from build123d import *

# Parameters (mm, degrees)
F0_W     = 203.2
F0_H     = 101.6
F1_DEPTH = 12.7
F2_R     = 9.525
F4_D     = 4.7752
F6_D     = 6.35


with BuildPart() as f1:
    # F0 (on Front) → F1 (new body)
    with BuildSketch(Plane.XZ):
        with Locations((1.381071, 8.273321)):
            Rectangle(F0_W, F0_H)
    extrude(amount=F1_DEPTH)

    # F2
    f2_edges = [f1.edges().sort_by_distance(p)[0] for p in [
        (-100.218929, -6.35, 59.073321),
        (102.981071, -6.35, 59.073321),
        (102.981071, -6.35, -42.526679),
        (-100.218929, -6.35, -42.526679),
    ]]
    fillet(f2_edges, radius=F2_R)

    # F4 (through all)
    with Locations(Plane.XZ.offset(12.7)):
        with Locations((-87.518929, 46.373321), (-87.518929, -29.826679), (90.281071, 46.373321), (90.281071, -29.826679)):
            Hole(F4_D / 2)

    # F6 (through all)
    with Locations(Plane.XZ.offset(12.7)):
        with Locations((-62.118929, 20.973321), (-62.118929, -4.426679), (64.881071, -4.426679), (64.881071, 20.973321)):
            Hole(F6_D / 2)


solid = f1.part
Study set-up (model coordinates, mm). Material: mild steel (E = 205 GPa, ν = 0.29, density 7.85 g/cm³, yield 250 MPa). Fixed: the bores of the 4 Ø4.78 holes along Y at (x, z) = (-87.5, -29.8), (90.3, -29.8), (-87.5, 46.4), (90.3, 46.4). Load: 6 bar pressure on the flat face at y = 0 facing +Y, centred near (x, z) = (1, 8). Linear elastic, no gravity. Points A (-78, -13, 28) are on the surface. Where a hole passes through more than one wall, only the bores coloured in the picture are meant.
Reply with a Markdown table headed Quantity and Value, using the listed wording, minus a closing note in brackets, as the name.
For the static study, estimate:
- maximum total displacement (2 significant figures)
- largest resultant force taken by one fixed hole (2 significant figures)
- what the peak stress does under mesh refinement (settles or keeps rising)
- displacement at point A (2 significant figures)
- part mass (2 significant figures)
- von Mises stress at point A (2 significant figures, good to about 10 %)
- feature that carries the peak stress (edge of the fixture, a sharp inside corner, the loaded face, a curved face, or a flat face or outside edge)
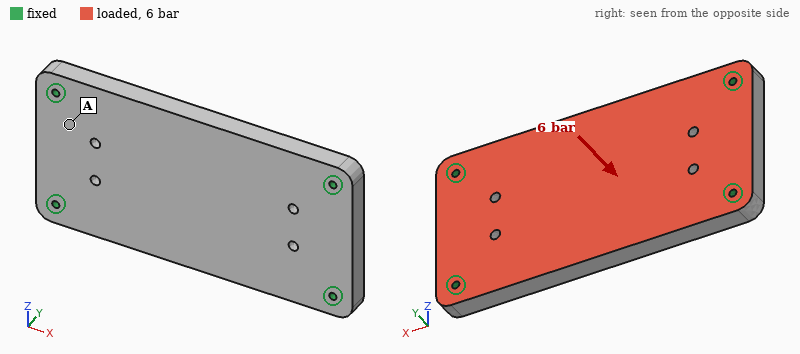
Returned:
| Quantity | Value |
|---|---|
| maximum total displacement | 69 µm |
| largest resultant force taken by one fixed hole | 3.1 kN |
| what the peak stress does under mesh refinement | keeps rising |
| displacement at point A | 11 µm |
| part mass | 2.0 kg |
| von Mises stress at point A | 22 MPa |
| feature that carries the peak stress | edge of the fixture |
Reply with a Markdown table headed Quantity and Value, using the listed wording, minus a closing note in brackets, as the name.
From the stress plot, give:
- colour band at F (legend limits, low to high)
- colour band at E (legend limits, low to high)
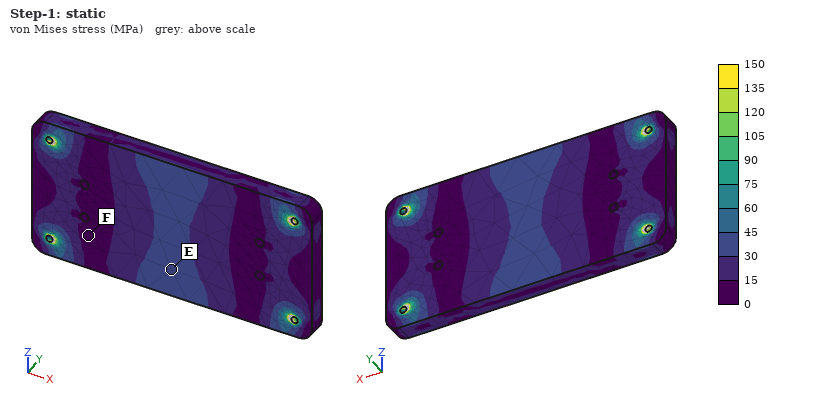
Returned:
| Quantity | Value |
|---|---|
| colour band at F | 0 to 15 MPa |
| colour band at E | 30 to 45 MPa |
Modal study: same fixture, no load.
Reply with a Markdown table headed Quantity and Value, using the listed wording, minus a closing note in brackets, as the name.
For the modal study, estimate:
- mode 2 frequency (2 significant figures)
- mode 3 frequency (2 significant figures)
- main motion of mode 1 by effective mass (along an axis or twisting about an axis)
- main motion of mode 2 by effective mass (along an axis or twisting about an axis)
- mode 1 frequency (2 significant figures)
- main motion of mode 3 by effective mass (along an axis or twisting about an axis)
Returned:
| Quantity | Value |
|---|---|
| mode 2 frequency | 2900 Hz |
| mode 3 frequency | 4600 Hz |
| main motion of mode 1 by effective mass | along Y |
| main motion of mode 2 by effective mass | twisting about X |
| mode 1 frequency | 1700 Hz |
| main motion of mode 3 by effective mass | twisting about Z |
